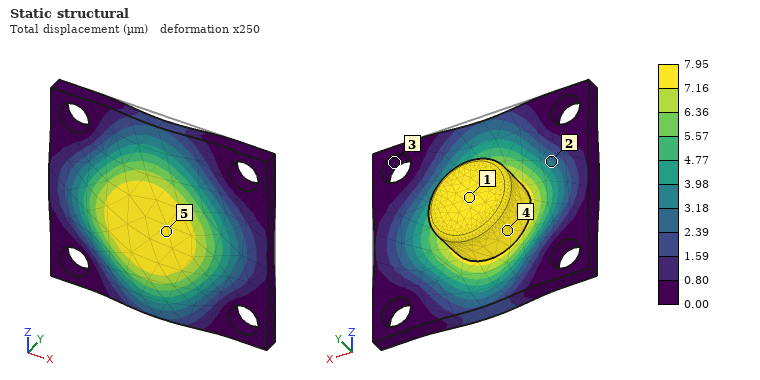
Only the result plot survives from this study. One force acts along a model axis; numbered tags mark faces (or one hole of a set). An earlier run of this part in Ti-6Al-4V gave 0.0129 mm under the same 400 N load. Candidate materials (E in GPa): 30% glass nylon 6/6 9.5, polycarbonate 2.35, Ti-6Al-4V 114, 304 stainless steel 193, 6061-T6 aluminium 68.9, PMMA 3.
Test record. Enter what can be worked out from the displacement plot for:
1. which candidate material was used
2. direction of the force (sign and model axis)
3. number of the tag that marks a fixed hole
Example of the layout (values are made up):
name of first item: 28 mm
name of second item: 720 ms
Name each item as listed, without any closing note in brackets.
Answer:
which candidate material was used: 304 stainless steel
direction of the force: -Y
number of the tag that marks a fixed hole: 3
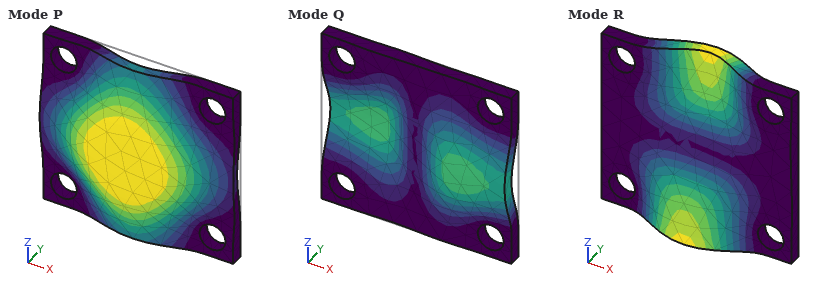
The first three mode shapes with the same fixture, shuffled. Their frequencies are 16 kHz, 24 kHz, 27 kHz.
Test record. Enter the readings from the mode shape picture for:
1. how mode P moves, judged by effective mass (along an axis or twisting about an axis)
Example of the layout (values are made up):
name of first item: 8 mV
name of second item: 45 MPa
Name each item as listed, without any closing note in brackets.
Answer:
how mode P moves, judged by effective mass: along Y
